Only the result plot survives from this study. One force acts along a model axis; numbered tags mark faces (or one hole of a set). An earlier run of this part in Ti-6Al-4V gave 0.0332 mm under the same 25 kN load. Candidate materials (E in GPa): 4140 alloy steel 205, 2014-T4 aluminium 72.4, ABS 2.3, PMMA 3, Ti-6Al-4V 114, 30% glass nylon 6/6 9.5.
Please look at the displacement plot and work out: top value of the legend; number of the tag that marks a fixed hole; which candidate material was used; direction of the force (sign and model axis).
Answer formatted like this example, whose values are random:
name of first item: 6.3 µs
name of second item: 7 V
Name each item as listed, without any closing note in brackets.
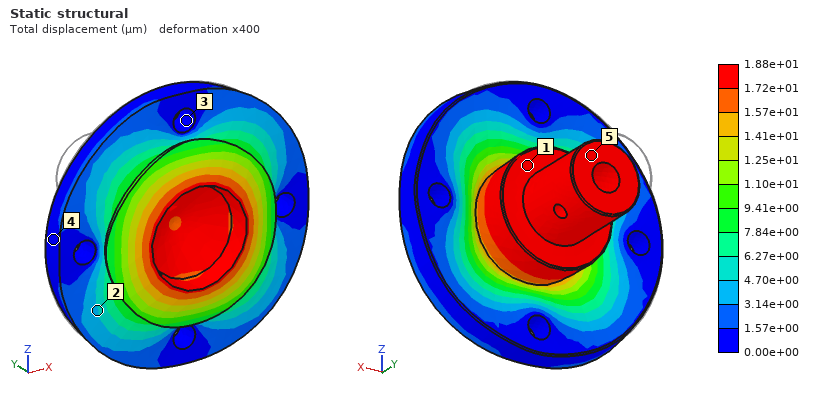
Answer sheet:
top value of the legend: 1.88e+01 µm
number of the tag that marks a fixed hole: 3
which candidate material was used: 4140 alloy steel
direction of the force: -Y
